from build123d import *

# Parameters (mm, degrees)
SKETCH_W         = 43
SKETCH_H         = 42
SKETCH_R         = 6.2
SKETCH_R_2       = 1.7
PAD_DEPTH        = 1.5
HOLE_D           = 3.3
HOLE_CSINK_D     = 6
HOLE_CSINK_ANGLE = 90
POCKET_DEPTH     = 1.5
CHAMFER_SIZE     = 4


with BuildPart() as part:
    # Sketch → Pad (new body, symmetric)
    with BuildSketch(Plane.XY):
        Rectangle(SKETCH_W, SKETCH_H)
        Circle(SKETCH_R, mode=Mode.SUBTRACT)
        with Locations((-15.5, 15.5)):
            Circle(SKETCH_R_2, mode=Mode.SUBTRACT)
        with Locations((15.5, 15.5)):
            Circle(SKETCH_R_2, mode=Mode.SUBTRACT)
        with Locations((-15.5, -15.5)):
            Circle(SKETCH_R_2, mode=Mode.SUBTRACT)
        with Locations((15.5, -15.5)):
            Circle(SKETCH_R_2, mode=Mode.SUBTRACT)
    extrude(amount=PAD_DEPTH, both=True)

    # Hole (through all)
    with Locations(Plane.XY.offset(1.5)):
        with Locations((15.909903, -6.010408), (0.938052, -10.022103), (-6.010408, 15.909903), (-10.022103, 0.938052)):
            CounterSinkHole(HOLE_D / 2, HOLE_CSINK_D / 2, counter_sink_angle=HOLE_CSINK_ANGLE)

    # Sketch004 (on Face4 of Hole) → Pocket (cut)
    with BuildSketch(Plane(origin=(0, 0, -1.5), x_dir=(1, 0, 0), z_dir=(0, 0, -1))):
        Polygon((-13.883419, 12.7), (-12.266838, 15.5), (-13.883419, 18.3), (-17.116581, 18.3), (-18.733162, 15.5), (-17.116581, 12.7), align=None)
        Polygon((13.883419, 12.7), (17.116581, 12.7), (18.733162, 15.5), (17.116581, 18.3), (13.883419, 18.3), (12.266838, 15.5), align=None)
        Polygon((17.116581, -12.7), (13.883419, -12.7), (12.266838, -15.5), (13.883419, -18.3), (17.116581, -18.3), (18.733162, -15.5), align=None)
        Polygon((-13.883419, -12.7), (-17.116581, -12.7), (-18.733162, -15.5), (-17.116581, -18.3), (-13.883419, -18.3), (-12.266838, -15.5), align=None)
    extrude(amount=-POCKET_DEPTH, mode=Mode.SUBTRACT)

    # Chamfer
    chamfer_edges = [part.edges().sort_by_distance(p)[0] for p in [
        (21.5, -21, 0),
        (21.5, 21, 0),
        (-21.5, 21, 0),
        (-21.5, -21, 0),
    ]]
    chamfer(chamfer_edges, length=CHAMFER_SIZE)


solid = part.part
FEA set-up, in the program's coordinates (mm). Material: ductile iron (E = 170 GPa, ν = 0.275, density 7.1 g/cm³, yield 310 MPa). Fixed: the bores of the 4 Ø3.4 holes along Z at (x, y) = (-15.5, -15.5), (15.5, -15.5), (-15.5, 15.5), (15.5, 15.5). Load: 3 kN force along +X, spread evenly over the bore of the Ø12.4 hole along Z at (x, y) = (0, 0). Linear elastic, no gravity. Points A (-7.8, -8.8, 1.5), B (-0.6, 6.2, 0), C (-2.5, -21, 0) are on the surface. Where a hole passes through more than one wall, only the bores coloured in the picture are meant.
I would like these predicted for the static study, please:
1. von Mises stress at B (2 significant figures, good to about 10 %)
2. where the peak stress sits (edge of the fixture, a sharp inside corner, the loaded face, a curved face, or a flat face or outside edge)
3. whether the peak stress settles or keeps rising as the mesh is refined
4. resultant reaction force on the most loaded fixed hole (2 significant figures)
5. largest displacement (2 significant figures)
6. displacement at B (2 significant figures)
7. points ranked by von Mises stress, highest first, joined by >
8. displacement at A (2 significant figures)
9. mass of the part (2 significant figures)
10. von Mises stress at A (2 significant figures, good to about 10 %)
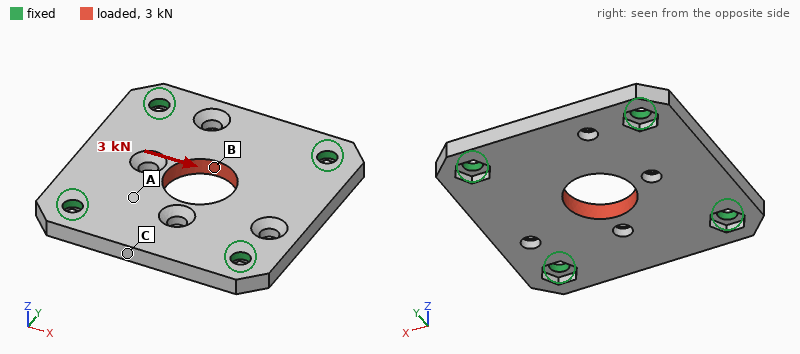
44 MPa
edge of the fixture
keeps rising
840 N
5.3 µm
3.6 µm
B > A > C
2.7 µm
33 g
27 MPa
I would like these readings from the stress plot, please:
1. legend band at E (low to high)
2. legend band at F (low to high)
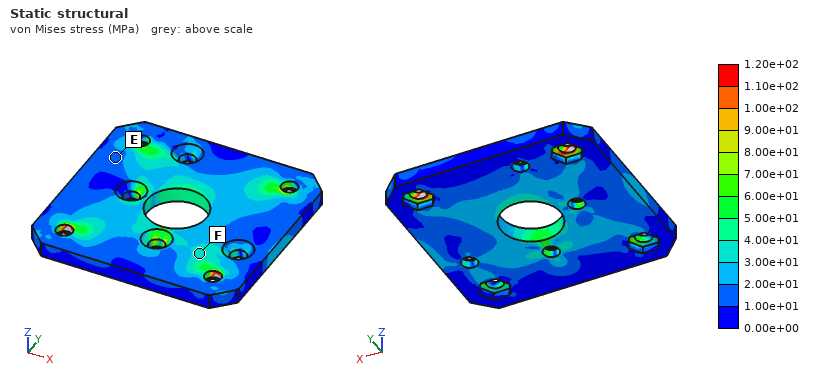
1.00e+01 to 2.00e+01 MPa
3.00e+01 to 4.00e+01 MPa
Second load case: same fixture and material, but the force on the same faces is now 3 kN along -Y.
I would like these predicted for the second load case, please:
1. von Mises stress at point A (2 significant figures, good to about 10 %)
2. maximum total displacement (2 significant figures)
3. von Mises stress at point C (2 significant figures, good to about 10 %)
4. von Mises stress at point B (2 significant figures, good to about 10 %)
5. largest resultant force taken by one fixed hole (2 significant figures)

27 MPa
5.4 µm
23 MPa
26 MPa
840 N
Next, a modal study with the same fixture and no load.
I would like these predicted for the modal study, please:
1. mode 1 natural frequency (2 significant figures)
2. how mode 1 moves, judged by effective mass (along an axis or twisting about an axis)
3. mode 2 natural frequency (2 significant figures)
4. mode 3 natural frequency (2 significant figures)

9600 Hz
along Z
13 kHz
13 kHz
